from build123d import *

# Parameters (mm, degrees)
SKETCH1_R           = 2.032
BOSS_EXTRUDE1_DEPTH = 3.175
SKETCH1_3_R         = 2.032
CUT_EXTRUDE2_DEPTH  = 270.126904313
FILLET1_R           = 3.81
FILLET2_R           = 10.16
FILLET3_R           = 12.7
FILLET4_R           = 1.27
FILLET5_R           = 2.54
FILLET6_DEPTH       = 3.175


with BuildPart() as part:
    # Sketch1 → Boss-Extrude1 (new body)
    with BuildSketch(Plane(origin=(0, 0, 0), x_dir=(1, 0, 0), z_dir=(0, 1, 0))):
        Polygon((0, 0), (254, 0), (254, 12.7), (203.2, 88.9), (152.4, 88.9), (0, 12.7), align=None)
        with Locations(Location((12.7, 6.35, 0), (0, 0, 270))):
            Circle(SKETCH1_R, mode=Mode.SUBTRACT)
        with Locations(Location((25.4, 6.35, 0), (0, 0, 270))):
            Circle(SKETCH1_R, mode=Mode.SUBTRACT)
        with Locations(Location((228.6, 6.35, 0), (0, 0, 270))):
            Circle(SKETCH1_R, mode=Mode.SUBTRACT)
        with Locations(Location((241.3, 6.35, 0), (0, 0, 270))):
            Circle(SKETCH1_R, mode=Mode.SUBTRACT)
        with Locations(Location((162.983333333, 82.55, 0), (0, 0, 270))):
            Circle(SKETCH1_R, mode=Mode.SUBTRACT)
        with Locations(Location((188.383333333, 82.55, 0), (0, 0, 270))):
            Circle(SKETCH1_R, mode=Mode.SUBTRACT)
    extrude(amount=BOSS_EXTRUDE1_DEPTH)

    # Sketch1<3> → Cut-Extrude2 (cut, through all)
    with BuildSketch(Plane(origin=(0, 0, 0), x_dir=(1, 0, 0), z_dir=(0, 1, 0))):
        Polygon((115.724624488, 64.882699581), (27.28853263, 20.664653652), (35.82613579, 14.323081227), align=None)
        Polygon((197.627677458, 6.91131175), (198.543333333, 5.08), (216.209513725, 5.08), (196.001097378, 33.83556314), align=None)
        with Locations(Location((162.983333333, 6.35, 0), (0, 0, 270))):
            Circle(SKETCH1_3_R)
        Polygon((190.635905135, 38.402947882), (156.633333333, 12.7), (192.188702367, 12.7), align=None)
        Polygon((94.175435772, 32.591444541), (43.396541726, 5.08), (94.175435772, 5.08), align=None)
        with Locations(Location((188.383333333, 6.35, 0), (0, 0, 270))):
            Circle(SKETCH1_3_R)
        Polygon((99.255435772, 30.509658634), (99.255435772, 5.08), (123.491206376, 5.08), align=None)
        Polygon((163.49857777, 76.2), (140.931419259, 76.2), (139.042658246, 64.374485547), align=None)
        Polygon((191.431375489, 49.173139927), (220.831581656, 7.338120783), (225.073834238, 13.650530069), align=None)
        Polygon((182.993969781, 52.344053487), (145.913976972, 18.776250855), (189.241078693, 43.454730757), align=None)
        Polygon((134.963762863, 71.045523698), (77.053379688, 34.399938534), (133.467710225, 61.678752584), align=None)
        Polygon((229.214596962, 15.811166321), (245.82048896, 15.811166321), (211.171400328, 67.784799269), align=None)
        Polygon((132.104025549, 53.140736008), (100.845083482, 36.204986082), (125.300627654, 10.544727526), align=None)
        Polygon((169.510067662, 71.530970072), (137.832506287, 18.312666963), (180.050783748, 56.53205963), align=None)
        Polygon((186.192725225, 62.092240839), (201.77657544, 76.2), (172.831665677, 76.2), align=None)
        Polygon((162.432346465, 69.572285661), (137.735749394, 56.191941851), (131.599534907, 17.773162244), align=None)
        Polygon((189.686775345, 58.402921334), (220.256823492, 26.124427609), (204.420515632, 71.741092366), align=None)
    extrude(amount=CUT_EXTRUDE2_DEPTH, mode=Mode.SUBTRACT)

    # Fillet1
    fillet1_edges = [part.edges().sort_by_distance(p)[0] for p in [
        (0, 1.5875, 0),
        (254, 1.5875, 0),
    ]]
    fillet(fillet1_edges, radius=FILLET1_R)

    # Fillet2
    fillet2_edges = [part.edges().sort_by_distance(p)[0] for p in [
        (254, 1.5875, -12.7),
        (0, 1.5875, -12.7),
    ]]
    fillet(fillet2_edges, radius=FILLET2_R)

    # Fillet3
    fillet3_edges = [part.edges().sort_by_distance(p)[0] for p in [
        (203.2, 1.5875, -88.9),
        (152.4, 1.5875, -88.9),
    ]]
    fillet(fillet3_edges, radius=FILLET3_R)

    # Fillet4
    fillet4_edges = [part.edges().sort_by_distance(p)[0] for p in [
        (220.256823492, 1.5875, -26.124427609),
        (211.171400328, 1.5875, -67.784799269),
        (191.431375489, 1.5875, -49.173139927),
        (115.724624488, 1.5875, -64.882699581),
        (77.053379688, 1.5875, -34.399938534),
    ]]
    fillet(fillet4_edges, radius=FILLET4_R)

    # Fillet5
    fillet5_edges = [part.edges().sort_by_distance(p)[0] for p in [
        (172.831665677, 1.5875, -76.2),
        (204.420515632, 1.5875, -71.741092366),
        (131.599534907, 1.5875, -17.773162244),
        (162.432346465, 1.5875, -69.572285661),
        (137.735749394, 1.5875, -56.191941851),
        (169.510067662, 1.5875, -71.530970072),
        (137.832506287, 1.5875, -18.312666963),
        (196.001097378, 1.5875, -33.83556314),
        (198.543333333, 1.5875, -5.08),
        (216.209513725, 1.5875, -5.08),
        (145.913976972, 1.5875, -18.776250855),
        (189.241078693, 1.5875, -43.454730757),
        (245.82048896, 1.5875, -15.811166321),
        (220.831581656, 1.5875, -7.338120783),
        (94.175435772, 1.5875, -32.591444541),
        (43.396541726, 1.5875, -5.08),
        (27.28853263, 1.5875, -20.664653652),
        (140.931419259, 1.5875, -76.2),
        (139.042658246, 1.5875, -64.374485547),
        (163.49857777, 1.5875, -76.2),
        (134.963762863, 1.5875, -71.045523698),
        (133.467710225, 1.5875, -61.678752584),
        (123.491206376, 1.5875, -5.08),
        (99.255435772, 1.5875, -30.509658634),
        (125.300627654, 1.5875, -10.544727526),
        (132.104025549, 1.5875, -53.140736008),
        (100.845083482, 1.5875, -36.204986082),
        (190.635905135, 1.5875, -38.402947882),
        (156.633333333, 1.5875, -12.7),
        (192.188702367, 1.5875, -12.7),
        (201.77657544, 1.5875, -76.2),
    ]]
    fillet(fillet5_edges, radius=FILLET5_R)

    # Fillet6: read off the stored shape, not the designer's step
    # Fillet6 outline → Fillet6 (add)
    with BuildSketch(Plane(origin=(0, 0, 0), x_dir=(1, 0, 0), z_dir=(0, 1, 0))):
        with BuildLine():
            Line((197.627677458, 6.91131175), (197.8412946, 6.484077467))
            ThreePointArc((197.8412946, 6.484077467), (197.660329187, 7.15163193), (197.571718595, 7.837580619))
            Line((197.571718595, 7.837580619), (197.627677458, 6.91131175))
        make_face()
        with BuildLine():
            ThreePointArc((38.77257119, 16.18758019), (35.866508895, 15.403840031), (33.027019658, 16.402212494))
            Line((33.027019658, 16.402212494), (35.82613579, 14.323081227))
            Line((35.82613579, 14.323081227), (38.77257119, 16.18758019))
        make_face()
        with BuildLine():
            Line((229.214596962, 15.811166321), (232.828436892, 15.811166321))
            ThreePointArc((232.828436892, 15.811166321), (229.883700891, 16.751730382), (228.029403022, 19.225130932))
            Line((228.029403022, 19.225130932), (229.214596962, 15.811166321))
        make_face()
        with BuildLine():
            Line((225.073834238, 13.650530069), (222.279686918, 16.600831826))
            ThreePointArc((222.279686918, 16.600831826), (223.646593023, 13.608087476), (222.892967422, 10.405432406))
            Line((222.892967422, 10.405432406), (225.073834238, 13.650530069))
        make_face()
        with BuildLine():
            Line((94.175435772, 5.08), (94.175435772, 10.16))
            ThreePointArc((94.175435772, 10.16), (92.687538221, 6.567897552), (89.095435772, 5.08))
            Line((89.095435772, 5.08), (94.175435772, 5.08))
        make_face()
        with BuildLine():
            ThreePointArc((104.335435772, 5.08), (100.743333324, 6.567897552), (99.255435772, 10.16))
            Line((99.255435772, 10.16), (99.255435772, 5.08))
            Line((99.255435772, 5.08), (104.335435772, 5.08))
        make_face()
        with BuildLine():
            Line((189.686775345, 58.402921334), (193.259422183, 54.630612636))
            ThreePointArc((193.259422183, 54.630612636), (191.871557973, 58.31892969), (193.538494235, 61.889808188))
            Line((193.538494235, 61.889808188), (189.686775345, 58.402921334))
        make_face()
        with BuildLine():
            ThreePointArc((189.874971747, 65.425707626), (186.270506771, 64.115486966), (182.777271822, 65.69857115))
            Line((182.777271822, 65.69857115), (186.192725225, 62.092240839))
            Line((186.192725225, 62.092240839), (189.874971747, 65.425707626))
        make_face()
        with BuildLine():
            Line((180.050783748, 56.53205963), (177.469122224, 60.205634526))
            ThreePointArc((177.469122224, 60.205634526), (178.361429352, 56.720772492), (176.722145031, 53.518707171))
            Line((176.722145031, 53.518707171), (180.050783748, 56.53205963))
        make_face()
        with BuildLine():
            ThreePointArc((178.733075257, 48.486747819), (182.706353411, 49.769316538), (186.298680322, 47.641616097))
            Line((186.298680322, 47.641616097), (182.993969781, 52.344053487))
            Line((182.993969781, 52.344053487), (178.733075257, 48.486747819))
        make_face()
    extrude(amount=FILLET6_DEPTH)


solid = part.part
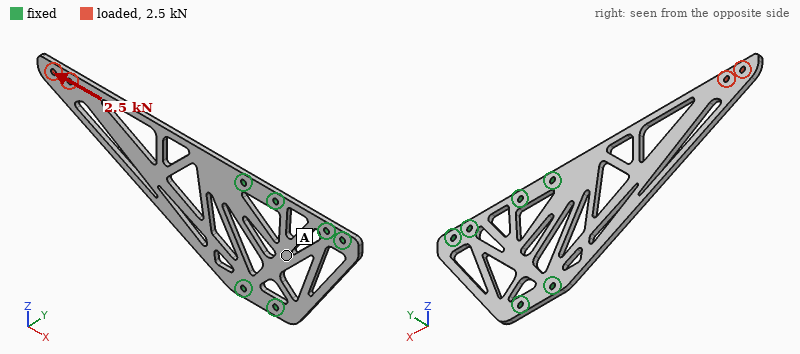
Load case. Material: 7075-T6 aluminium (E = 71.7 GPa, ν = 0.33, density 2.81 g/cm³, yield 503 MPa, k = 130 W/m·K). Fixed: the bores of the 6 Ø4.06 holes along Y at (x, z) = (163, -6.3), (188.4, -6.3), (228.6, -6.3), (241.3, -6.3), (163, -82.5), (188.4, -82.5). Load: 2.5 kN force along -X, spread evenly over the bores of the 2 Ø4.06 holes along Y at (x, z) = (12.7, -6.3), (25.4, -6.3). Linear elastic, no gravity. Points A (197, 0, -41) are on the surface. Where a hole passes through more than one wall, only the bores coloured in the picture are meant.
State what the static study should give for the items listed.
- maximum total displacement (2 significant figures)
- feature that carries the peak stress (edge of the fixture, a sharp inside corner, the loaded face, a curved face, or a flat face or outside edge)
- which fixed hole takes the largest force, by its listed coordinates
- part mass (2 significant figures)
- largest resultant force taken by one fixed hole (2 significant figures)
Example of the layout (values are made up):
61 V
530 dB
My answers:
0.42 mm
a curved face
(163, -6.3)
84 g
2.3 kN
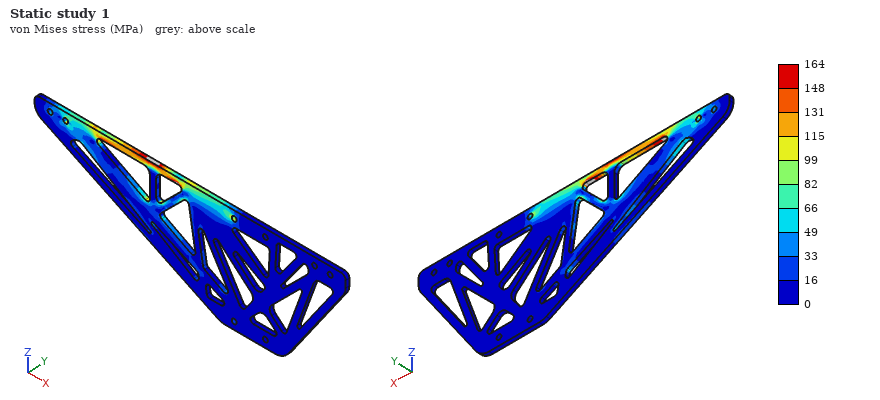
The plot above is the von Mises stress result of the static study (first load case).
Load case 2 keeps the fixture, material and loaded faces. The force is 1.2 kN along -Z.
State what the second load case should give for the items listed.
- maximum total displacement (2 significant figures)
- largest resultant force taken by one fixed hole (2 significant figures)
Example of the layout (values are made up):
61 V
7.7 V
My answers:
0.58 mm
2.2 kN
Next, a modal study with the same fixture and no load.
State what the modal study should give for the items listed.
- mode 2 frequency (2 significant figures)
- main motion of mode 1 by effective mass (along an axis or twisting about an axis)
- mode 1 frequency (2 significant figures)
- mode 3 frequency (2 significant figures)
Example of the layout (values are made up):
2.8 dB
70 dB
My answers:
580 Hz
along Y
120 Hz
900 Hz
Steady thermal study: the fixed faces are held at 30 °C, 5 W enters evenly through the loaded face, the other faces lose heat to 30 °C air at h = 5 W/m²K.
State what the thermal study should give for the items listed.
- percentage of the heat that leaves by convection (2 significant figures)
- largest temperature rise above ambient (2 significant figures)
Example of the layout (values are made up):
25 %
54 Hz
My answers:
30 %
57 K
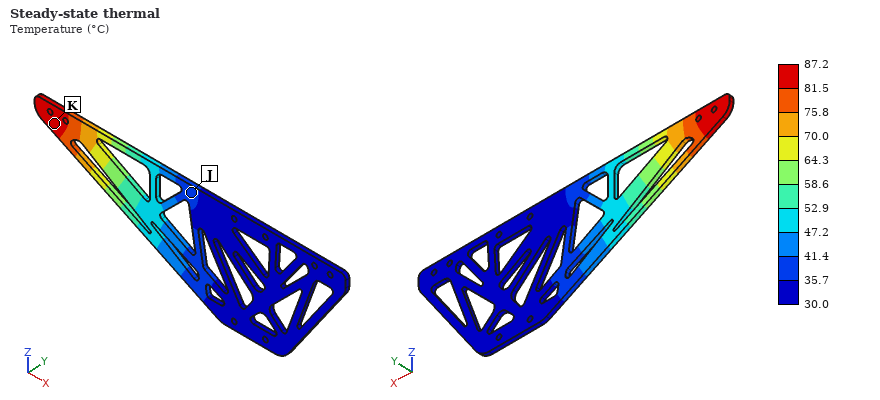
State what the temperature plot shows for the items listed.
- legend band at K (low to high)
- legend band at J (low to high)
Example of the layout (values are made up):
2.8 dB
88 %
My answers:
81.5 to 87.2 °C
35.7 to 41.4 °C
